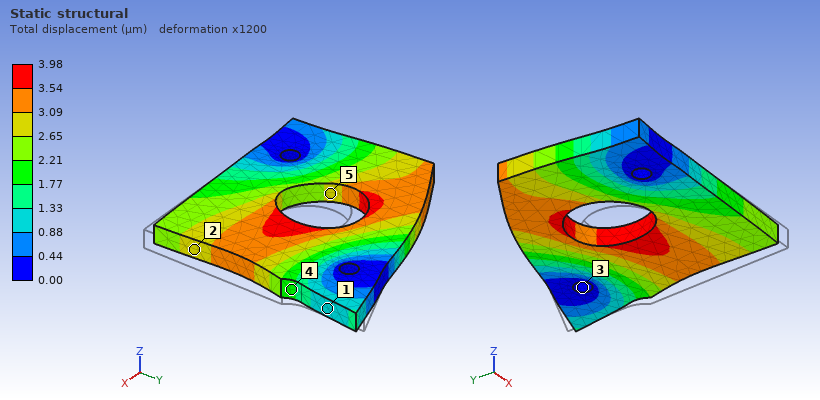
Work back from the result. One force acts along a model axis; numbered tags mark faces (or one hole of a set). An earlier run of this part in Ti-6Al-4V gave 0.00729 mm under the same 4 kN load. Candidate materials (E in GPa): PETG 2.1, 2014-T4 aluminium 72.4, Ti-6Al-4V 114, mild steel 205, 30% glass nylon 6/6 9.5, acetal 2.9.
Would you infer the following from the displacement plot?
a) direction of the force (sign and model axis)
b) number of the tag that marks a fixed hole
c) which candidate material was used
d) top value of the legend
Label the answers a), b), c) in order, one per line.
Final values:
a) -X
b) 3
c) mild steel
d) 3.98 µm
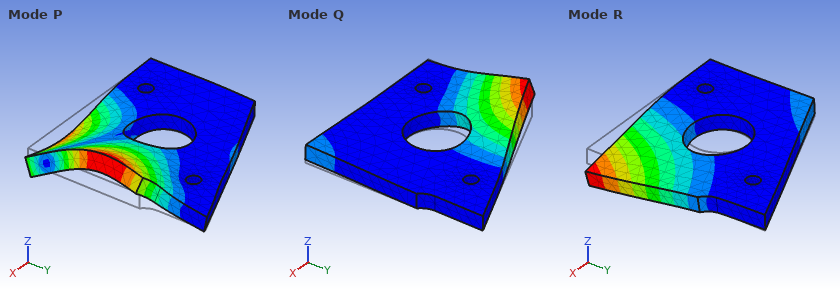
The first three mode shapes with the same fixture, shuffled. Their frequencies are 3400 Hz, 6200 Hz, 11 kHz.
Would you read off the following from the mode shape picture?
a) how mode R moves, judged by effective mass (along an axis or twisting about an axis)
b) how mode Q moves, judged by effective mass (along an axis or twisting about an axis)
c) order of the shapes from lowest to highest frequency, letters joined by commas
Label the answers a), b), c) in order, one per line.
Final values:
a) along Z
b) along Z
c) R, Q, P
